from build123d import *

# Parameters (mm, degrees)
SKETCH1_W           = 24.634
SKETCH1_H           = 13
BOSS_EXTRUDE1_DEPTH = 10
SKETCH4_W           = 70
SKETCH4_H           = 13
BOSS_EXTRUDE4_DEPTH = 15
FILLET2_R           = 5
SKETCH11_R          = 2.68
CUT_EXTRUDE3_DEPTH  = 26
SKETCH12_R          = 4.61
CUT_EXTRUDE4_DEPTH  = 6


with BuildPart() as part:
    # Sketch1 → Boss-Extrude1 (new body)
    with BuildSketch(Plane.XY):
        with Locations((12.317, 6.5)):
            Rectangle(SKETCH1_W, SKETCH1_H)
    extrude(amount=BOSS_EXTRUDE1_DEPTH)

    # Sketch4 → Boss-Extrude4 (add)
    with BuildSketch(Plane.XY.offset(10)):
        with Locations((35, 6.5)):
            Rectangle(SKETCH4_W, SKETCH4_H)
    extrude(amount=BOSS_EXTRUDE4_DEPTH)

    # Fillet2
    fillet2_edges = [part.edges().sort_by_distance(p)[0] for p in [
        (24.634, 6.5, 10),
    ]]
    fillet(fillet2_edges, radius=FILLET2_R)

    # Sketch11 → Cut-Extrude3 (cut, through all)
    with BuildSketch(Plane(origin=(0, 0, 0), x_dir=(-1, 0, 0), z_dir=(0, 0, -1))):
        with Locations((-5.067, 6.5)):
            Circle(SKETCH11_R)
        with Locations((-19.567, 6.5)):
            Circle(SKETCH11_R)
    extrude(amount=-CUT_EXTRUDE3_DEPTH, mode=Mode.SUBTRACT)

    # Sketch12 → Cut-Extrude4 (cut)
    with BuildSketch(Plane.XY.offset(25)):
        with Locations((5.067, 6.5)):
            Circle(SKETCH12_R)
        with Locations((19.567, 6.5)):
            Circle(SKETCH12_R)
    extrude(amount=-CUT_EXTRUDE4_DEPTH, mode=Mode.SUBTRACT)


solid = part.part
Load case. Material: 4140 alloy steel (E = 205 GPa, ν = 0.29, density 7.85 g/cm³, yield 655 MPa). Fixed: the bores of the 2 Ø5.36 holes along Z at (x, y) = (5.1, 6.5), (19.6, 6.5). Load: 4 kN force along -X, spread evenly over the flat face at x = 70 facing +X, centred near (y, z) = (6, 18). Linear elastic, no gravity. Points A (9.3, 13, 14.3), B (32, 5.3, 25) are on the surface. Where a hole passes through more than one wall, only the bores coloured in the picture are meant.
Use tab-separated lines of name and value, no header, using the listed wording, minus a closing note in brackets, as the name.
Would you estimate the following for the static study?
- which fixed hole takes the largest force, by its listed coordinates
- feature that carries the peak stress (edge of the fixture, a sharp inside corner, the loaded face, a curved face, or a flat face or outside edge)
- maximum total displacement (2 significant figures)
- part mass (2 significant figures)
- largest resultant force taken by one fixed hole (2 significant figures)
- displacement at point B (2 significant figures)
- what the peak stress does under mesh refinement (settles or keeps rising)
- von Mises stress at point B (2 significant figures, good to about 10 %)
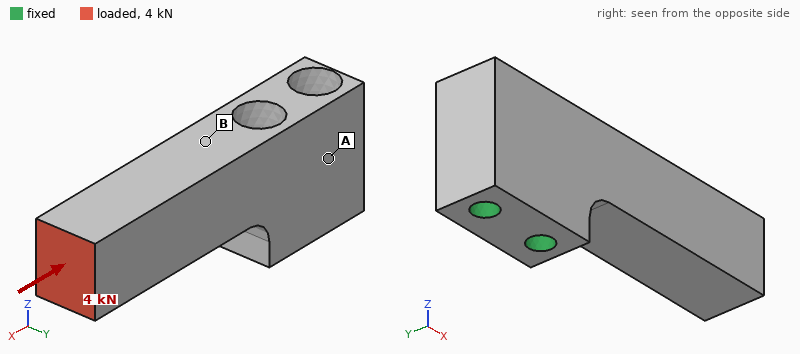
which fixed hole takes the largest force, by its listed coordinates	(19.6, 6.5)
feature that carries the peak stress	edge of the fixture
maximum total displacement	11 µm
part mass	120 g
largest resultant force taken by one fixed hole	3.4 kN
displacement at point B	3.9 µm
what the peak stress does under mesh refinement	keeps rising
von Mises stress at point B	16 MPa
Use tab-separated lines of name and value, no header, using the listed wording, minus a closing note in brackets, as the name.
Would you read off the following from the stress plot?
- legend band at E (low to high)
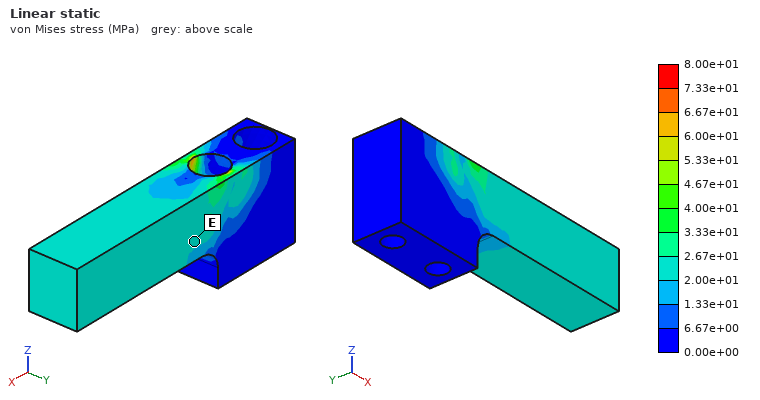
legend band at E	2.00e+01 to 2.67e+01 MPa
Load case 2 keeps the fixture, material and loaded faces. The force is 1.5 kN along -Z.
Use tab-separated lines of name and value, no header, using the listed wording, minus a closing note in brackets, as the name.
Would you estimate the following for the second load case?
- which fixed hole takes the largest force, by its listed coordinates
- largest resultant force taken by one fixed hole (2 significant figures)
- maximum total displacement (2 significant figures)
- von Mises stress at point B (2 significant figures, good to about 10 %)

which fixed hole takes the largest force, by its listed coordinates	(19.6, 6.5)
largest resultant force taken by one fixed hole	2.9 kN
maximum total displacement	0.10 mm
von Mises stress at point B	96 MPa
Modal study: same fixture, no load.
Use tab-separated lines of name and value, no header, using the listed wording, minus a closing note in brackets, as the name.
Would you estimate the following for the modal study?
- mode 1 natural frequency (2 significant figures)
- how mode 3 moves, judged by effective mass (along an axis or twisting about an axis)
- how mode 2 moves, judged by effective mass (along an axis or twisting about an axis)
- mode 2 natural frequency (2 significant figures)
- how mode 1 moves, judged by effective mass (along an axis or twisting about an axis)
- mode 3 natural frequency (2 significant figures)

mode 1 natural frequency	3700 Hz
how mode 3 moves, judged by effective mass	twisting about X
how mode 2 moves, judged by effective mass	along Z
mode 2 natural frequency	4300 Hz
how mode 1 moves, judged by effective mass	along Y
mode 3 natural frequency	14 kHz
